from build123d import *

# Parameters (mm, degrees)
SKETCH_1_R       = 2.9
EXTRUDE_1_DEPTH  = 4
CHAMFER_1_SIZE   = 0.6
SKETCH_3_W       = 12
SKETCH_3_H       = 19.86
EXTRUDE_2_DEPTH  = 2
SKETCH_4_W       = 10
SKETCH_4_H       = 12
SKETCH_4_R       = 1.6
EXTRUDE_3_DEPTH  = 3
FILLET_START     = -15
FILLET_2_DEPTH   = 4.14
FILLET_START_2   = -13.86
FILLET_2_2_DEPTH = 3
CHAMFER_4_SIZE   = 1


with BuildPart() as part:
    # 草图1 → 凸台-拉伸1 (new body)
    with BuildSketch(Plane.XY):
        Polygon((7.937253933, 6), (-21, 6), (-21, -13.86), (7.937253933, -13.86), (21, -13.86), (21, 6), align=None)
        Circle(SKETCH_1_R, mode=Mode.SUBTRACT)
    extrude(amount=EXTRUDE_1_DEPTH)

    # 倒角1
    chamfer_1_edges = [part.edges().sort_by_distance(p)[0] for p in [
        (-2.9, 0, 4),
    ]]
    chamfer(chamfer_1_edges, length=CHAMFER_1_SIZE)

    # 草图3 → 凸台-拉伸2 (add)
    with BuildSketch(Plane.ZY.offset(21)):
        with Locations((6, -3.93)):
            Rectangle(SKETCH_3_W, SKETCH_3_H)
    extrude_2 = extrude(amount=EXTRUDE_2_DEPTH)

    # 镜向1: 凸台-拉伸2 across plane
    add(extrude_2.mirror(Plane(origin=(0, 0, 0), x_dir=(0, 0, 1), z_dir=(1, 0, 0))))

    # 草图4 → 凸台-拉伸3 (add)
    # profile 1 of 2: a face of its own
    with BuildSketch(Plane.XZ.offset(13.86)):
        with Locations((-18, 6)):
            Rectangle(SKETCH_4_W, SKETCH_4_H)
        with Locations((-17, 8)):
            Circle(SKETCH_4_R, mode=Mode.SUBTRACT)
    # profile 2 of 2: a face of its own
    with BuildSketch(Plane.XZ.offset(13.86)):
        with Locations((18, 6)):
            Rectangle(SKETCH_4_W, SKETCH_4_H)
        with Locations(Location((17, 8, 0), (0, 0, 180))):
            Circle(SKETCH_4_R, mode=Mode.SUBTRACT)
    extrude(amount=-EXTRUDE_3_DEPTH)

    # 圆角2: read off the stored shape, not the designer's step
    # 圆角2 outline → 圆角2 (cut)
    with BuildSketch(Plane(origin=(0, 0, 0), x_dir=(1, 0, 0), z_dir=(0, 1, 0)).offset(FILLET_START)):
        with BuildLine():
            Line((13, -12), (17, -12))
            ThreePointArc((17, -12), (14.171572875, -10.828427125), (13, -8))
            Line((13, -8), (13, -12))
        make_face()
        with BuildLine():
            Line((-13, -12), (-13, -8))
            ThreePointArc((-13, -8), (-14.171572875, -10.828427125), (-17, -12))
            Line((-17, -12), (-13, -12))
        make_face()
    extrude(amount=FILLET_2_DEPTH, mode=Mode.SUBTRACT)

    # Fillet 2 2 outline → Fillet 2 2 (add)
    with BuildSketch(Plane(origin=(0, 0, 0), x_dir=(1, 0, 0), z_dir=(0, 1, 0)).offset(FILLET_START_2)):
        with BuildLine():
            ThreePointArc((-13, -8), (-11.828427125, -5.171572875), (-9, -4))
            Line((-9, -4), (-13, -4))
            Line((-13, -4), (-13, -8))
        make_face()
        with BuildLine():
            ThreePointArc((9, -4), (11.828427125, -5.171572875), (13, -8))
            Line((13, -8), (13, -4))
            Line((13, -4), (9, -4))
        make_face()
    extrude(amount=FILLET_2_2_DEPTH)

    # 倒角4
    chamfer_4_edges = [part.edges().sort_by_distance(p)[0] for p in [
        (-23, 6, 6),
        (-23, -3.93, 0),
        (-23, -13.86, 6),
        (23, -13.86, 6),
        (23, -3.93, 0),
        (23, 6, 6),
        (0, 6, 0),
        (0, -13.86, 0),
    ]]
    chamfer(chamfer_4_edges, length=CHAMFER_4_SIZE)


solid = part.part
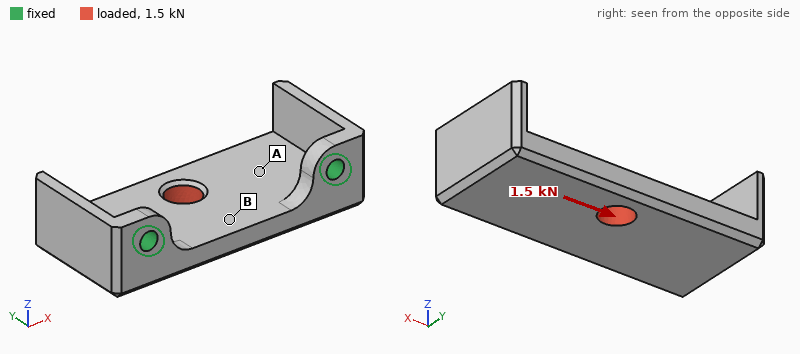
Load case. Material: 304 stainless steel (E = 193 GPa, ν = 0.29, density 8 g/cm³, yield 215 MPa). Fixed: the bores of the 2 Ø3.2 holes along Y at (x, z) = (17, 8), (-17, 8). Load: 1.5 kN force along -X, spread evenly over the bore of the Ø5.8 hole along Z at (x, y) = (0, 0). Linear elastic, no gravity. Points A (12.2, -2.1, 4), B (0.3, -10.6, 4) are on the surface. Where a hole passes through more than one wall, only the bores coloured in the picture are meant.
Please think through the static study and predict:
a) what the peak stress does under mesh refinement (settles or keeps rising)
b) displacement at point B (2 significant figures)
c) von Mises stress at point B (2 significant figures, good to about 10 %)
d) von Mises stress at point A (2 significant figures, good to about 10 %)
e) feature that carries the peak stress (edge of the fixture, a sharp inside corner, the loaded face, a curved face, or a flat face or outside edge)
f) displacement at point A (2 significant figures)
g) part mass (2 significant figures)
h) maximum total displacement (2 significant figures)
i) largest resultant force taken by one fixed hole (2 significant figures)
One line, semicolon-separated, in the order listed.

keeps rising; 5.1 µm; 14 MPa; 30 MPa; edge of the fixture; 8.3 µm; 35 g; 13 µm; 910 N
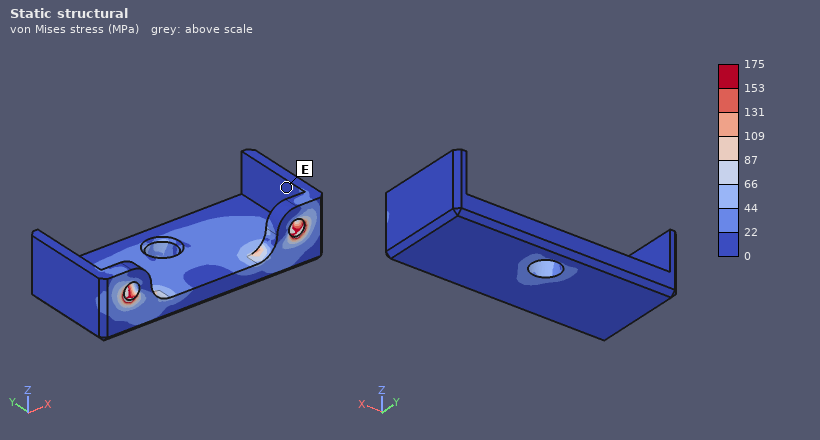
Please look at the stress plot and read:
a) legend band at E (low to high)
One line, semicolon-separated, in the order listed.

0 to 22 MPa
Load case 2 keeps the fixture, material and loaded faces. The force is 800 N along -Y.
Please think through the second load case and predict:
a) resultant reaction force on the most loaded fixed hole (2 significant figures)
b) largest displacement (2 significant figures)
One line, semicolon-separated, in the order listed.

410 N; 20 µm
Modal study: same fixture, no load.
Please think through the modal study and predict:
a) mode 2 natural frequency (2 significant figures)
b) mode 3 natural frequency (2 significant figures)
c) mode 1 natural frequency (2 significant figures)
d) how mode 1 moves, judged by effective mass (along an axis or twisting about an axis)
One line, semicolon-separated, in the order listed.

8200 Hz; 13 kHz; 4700 Hz; along Z
